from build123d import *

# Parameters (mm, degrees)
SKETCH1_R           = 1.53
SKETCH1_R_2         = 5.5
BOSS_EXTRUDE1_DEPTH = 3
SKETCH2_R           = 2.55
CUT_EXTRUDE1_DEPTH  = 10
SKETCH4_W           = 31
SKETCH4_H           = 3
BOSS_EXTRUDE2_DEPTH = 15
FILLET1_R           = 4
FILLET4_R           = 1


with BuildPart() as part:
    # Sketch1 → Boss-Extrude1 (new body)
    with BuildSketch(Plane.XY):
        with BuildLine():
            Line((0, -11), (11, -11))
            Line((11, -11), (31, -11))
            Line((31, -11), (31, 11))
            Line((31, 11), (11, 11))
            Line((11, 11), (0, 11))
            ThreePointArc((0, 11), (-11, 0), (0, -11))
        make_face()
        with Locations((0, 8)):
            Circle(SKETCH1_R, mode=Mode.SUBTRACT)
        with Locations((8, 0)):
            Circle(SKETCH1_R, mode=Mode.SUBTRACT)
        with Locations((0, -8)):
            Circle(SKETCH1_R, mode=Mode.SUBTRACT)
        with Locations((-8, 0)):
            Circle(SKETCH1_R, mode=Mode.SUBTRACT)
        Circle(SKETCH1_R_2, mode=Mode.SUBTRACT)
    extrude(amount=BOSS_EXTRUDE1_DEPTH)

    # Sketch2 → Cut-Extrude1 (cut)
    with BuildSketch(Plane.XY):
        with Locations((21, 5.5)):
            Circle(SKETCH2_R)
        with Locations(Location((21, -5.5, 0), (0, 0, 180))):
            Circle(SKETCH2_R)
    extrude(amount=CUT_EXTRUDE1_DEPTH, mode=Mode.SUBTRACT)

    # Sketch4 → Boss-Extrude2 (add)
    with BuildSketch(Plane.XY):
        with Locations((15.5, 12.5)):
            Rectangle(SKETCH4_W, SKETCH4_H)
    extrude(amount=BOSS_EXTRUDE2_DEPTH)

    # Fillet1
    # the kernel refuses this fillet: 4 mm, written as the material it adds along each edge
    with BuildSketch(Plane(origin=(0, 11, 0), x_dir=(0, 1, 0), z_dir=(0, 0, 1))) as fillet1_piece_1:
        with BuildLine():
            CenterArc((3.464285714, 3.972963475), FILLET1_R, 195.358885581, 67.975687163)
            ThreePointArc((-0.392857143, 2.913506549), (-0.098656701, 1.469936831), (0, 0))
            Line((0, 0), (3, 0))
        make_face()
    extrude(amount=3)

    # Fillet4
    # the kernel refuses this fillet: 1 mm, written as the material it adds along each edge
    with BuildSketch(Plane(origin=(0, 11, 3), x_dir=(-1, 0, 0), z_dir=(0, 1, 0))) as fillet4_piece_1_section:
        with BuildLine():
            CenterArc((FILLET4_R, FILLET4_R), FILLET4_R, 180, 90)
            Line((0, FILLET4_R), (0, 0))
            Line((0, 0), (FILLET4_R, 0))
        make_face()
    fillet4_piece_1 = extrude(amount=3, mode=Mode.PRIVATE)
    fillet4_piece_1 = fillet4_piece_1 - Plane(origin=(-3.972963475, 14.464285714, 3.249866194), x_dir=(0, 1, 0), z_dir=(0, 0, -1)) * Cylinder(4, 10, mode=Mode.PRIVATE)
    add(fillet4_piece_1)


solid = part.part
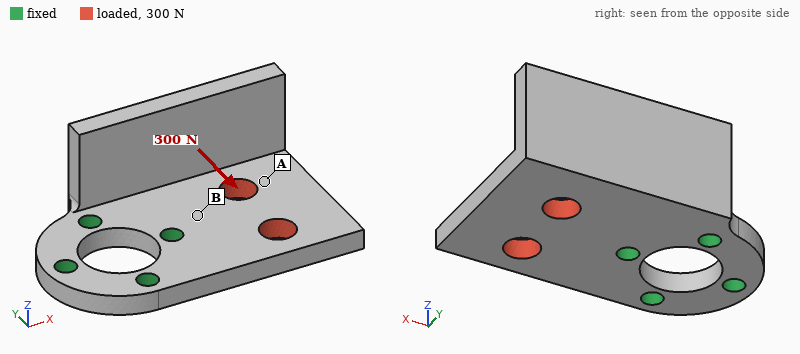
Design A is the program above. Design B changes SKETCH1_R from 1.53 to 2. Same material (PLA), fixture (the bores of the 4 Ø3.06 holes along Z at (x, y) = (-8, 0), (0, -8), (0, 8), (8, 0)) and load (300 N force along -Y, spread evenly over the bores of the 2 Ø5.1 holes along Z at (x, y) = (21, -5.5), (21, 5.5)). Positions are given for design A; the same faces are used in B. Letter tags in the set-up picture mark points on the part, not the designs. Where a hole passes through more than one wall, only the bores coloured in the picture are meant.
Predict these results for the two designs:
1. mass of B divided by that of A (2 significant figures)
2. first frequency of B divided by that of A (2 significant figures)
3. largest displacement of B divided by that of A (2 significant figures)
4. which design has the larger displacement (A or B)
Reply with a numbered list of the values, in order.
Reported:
1. 0.98
2. 1.1
3. 0.92
4. A
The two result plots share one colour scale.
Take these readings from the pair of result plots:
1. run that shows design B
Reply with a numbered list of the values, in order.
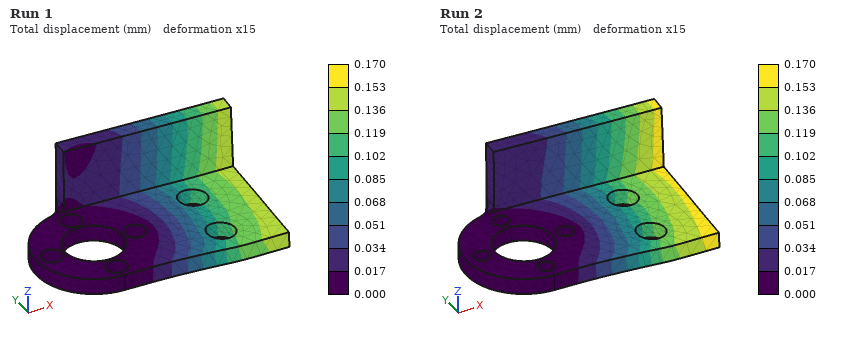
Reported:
1. Run 1
